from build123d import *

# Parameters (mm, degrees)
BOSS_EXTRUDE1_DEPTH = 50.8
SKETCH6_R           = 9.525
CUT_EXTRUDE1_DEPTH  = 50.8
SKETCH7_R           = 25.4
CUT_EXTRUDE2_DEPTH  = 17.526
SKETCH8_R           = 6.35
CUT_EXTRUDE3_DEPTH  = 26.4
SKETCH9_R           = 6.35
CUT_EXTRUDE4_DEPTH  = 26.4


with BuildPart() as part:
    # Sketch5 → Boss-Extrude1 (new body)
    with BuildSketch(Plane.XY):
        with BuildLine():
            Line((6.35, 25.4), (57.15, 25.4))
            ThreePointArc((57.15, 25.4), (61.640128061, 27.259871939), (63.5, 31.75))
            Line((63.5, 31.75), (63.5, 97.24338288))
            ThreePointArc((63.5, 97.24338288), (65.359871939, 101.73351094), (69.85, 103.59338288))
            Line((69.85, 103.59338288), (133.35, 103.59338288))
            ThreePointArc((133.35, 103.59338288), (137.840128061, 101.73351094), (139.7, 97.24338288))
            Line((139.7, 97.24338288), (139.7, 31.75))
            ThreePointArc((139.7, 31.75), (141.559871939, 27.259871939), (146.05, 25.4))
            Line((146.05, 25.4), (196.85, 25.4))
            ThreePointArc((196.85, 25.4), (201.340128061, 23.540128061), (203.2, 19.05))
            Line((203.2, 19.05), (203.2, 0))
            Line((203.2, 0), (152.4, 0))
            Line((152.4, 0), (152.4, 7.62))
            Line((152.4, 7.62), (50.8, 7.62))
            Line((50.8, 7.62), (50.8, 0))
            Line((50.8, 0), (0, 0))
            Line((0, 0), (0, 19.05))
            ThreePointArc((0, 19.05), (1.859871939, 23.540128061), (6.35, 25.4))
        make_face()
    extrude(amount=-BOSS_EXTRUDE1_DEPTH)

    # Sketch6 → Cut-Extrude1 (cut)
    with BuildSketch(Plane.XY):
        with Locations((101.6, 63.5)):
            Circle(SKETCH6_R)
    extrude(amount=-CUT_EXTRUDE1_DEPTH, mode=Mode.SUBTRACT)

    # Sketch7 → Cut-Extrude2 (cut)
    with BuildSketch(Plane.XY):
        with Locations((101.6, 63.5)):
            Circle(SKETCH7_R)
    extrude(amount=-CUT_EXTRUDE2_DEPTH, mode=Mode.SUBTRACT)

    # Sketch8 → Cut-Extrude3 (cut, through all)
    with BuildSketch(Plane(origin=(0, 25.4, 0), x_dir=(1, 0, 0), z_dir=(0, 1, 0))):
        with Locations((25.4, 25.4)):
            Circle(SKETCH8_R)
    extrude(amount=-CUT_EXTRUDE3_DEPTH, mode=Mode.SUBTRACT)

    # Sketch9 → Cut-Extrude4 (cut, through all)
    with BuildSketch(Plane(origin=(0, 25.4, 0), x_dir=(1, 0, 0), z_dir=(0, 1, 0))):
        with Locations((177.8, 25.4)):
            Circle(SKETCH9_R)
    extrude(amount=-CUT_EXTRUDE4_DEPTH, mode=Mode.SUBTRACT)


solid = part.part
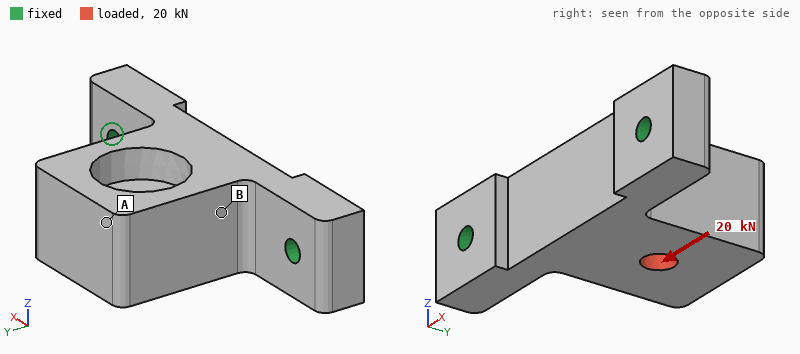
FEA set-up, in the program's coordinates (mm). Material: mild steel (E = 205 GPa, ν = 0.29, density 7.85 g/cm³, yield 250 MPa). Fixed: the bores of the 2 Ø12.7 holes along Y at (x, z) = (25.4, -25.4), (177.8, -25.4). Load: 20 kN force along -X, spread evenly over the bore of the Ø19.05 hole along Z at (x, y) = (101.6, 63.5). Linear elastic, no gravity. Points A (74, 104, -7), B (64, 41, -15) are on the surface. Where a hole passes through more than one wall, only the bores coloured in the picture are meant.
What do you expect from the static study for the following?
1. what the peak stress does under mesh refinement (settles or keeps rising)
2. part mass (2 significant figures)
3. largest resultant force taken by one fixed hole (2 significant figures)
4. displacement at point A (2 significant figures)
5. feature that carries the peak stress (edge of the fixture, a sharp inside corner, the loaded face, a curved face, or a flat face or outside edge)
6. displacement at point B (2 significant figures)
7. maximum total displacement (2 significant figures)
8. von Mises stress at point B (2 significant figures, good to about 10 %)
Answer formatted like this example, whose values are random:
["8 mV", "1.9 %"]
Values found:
["keeps rising", "3.7 kg", "13 kN", "27 µm", "edge of the fixture", "12 µm", "29 µm", "16 MPa"]
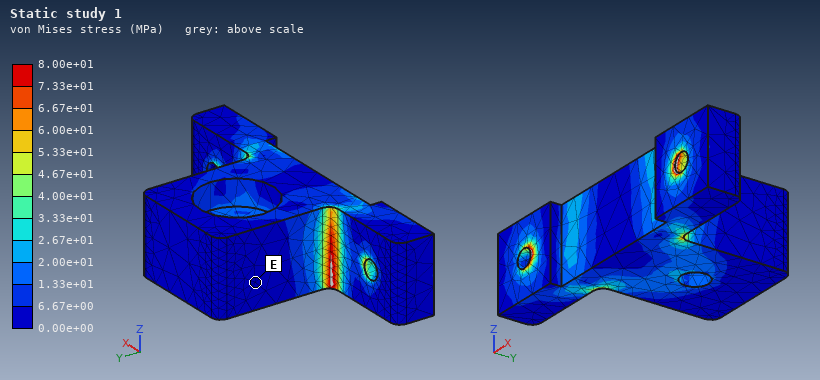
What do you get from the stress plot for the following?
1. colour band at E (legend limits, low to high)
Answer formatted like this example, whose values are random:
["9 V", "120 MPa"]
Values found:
["0.00e+00 to 6.67e+00 MPa"]
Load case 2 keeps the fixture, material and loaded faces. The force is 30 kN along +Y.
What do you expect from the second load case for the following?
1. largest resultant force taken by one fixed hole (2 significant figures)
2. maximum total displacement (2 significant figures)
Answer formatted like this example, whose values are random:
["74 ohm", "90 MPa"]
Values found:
["18 kN", "60 µm"]
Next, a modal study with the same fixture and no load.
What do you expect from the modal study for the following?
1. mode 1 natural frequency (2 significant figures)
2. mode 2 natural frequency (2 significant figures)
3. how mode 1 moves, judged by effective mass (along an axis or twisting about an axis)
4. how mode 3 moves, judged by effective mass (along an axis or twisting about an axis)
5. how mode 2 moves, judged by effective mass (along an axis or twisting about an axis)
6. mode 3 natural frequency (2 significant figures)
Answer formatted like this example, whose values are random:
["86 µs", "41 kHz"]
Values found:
["1300 Hz", "3200 Hz", "along Z", "along Y", "along X", "3500 Hz"]
